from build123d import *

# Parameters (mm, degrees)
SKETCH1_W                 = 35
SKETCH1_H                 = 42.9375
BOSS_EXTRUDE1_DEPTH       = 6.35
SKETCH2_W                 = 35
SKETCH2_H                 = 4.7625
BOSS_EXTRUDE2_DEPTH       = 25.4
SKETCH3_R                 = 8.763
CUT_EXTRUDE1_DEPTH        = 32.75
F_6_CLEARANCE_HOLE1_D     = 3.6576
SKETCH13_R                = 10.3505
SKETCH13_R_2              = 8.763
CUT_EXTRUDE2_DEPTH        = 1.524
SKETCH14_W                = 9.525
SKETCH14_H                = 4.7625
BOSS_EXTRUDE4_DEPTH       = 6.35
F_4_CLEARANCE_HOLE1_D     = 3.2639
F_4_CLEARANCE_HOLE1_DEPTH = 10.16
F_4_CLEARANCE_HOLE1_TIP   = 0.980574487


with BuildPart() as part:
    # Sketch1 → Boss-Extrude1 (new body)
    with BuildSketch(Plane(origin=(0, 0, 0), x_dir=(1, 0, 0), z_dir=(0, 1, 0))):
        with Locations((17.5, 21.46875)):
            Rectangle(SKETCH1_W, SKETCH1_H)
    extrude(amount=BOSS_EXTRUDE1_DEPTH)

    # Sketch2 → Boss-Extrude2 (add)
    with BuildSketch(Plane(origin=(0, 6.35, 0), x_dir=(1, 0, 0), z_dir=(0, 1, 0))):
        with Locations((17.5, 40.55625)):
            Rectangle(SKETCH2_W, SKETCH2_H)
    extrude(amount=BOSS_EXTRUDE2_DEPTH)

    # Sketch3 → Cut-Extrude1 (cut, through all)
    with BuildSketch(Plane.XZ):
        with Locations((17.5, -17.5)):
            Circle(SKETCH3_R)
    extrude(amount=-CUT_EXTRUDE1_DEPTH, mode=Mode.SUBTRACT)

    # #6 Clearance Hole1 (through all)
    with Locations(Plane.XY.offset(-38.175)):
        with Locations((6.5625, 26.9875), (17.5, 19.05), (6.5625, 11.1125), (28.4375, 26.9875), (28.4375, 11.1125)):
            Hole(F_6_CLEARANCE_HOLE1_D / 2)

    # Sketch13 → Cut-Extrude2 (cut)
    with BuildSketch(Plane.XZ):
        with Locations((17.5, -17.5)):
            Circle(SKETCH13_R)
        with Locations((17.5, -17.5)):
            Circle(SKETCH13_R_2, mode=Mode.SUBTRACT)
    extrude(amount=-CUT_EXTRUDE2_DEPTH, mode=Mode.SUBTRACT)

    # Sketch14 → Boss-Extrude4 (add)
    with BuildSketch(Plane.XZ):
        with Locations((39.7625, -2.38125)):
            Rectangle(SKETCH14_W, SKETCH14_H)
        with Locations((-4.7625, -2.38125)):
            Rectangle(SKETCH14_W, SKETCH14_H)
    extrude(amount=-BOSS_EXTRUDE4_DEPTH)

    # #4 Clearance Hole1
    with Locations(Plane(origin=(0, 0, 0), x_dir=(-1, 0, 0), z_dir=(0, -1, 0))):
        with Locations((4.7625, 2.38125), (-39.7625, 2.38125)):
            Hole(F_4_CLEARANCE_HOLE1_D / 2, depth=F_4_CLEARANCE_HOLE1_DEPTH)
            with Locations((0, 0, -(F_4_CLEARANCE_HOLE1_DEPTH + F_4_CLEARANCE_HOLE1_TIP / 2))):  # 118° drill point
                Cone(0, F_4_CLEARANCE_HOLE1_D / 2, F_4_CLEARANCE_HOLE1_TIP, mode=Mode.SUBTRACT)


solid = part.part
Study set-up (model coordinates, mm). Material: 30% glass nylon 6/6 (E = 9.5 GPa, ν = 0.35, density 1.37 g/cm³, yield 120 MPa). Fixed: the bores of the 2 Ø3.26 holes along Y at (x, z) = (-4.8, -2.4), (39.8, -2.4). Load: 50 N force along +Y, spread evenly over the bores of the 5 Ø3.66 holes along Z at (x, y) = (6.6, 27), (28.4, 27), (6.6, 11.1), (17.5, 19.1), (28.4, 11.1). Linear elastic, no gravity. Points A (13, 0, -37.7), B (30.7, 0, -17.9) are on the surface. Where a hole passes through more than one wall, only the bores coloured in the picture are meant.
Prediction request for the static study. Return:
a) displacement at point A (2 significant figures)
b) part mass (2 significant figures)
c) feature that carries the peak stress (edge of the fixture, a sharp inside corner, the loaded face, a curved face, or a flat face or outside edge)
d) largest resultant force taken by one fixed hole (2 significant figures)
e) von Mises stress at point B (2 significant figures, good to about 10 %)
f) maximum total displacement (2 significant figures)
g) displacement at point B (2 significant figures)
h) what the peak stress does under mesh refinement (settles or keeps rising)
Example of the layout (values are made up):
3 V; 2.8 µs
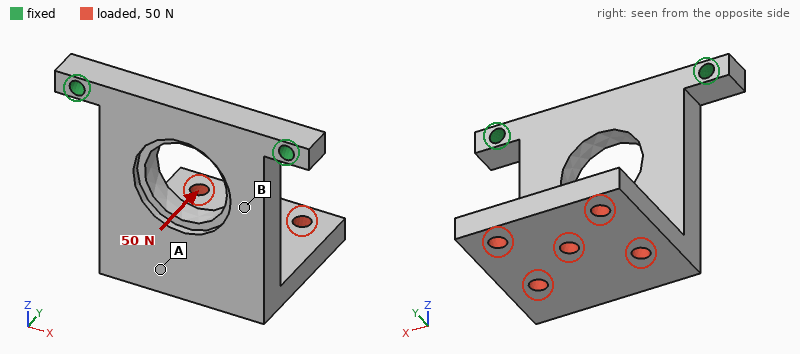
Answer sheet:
0.58 mm; 17 g; edge of the fixture; 25 N; 10 MPa; 0.87 mm; 0.22 mm; keeps rising
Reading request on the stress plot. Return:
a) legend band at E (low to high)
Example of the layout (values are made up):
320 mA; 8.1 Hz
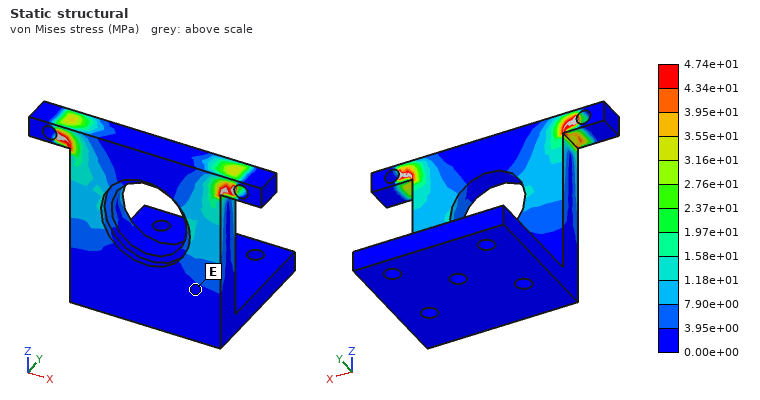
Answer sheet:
0.00e+00 to 3.95e+00 MPa
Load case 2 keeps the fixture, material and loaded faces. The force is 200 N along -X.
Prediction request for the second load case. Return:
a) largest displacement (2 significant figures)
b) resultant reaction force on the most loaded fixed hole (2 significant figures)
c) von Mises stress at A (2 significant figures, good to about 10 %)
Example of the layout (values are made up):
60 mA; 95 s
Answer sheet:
0.60 mm; 240 N; 9.5 MPa
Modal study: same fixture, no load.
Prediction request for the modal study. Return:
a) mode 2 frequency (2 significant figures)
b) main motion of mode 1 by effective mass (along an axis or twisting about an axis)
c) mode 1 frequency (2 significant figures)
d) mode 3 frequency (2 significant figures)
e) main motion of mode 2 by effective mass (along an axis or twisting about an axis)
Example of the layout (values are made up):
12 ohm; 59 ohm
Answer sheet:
1300 Hz; along Y; 430 Hz; 1900 Hz; along X
